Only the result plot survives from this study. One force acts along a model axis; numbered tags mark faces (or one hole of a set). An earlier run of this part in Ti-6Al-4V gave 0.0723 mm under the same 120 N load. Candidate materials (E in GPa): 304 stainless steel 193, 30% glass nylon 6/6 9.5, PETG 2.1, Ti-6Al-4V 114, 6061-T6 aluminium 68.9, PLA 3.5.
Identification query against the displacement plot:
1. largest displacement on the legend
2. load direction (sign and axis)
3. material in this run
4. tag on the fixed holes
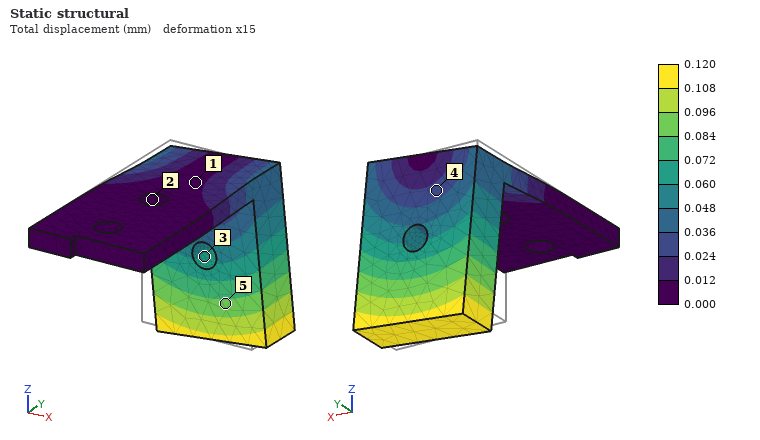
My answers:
0.120 mm
+X
6061-T6 aluminium
2
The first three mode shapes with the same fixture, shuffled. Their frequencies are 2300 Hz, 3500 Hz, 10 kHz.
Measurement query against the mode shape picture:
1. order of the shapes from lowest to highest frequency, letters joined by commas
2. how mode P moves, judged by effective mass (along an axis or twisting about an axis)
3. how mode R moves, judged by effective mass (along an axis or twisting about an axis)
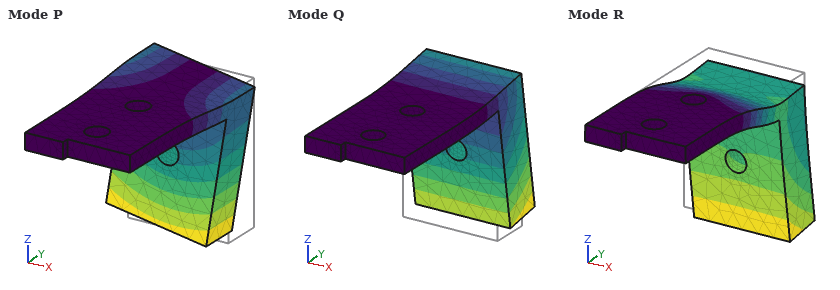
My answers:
Q, P, R
along X
along Z
